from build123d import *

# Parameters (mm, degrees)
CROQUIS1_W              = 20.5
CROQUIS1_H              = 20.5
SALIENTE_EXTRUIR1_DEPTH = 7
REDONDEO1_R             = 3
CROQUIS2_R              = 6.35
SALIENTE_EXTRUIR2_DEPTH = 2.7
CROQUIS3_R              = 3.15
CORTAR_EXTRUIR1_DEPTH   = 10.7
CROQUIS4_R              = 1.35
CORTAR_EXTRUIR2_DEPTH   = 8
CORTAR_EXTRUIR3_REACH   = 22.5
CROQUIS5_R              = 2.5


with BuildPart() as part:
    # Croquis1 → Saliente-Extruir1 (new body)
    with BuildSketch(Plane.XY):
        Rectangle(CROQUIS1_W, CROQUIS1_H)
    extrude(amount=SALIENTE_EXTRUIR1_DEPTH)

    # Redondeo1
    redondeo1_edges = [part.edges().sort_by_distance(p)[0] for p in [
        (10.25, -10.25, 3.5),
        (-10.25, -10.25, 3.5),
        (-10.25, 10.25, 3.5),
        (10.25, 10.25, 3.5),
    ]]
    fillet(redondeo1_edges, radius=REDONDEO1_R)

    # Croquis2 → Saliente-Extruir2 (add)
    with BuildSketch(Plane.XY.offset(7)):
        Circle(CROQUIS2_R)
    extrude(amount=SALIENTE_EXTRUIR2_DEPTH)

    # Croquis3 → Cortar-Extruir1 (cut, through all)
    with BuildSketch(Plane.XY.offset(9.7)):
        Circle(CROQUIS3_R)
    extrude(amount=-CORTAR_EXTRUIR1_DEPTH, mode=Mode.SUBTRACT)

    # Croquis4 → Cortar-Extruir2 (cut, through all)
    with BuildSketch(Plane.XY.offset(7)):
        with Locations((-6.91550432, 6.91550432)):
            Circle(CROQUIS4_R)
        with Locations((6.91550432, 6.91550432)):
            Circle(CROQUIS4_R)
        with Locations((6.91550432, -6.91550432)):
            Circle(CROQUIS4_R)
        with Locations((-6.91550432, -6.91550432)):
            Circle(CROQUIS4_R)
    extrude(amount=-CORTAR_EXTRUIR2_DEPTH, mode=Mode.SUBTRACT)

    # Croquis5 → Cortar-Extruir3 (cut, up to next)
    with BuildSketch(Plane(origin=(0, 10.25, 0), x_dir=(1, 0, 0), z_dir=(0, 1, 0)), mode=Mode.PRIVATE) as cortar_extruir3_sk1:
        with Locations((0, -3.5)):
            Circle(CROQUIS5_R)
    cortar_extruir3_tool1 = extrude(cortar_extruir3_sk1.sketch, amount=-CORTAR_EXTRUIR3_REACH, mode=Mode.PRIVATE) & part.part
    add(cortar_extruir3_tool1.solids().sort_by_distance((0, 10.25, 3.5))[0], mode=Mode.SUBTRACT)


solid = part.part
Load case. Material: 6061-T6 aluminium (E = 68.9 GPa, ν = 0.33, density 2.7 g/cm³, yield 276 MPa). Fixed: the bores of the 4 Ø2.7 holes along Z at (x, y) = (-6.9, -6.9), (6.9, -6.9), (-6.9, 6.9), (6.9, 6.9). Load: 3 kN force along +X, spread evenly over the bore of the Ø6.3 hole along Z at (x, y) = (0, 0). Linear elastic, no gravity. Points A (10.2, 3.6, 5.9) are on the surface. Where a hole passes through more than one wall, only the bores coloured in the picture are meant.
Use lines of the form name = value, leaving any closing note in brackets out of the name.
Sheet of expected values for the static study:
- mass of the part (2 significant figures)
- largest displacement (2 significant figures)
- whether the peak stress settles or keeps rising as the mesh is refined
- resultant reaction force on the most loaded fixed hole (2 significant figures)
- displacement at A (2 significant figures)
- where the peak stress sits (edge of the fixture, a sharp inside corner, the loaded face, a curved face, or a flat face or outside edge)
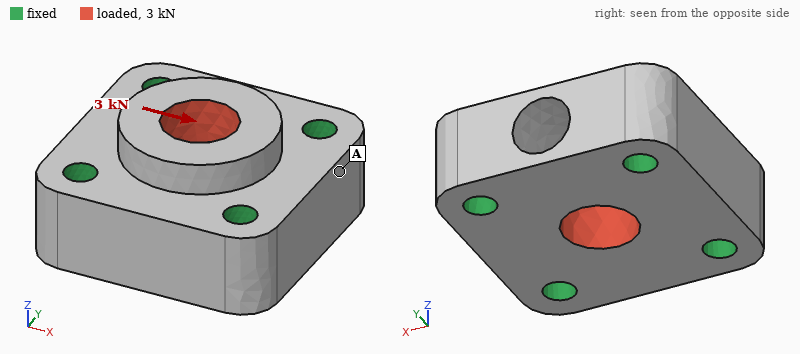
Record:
mass of the part = 7.1 g
largest displacement = 5.1 µm
whether the peak stress settles or keeps rising as the mesh is refined = keeps rising
resultant reaction force on the most loaded fixed hole = 940 N
displacement at A = 1.6 µm
where the peak stress sits = edge of the fixture
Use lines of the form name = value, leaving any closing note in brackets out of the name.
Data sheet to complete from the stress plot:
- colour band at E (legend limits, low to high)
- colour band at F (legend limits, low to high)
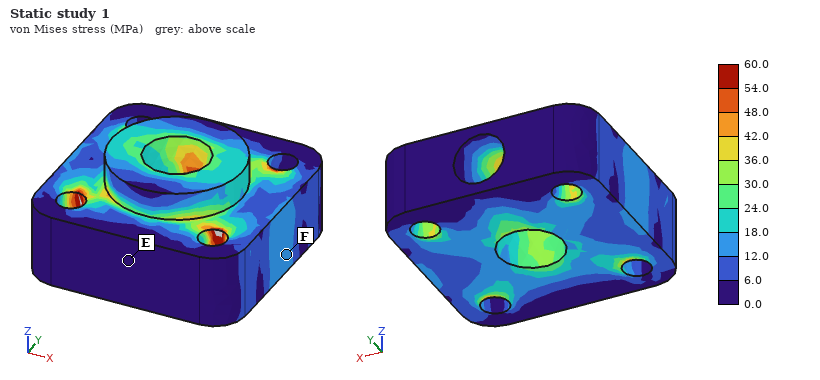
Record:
colour band at E = 0.0 to 6.0 MPa
colour band at F = 12.0 to 18.0 MPa
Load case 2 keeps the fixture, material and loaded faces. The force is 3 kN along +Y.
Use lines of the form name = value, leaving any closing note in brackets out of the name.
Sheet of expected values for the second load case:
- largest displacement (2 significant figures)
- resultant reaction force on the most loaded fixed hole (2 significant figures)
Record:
largest displacement = 4.8 µm
resultant reaction force on the most loaded fixed hole = 880 N
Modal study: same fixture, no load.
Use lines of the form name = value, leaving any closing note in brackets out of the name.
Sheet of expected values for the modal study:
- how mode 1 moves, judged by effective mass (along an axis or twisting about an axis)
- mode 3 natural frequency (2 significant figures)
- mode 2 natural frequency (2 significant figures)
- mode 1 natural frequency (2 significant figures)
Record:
how mode 1 moves, judged by effective mass = along Z
mode 3 natural frequency = 95 kHz
mode 2 natural frequency = 92 kHz
mode 1 natural frequency = 84 kHz
